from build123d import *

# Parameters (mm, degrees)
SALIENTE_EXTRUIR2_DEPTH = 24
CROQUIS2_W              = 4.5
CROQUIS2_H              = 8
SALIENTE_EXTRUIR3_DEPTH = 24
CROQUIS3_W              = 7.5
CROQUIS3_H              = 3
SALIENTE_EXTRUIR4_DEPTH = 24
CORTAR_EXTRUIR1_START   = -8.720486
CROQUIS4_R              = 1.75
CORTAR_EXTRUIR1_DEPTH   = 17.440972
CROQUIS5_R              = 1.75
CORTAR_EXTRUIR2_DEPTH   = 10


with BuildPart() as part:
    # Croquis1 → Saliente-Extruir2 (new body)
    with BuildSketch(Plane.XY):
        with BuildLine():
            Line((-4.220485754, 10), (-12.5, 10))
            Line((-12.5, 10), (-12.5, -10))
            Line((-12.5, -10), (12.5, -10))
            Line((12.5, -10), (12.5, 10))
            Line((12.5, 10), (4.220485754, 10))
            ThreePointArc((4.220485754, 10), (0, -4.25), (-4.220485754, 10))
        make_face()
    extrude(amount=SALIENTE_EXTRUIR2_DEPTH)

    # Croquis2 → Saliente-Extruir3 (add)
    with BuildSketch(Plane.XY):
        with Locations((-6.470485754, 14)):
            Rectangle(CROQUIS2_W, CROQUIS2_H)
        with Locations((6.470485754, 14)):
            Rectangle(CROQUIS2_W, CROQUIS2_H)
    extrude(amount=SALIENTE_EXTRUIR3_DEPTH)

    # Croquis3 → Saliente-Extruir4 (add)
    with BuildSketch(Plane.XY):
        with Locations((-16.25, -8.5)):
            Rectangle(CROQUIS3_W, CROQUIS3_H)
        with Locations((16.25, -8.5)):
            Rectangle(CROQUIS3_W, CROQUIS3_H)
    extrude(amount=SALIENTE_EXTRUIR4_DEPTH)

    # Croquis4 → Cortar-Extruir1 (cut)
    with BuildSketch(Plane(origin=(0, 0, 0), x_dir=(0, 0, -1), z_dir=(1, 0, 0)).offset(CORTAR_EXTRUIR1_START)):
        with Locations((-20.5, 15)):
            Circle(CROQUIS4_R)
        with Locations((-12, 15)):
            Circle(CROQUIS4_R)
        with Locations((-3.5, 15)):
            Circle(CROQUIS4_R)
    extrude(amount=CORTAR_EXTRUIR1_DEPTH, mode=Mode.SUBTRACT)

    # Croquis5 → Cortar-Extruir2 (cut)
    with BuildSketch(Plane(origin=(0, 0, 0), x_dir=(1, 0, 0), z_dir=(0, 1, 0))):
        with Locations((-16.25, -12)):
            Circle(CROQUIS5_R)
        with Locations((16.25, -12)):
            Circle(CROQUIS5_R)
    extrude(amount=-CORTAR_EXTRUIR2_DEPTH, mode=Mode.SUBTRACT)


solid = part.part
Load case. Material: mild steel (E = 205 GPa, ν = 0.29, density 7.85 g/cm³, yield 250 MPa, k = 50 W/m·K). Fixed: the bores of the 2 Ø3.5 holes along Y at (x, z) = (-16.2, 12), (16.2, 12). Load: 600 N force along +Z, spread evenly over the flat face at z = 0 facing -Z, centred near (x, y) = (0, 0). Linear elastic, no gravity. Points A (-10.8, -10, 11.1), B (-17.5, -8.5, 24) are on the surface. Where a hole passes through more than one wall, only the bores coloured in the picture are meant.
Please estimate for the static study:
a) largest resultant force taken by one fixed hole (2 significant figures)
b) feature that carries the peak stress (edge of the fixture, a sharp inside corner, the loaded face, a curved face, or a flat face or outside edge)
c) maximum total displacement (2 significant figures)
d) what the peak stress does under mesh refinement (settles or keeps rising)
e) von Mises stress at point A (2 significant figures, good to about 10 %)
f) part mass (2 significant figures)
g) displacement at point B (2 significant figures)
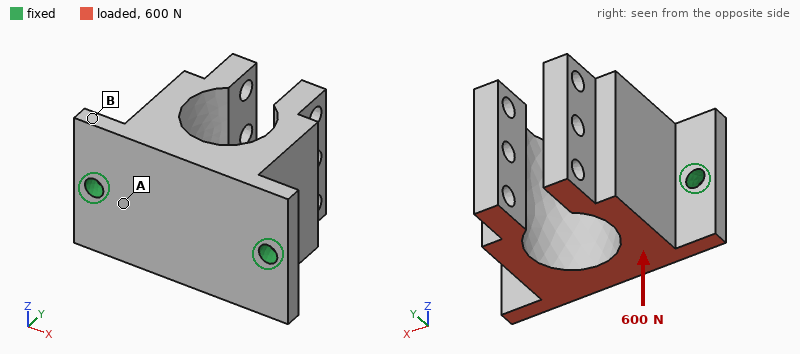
300 N
edge of the fixture
23 µm
keeps rising
17 MPa
80 g
7.4 µm
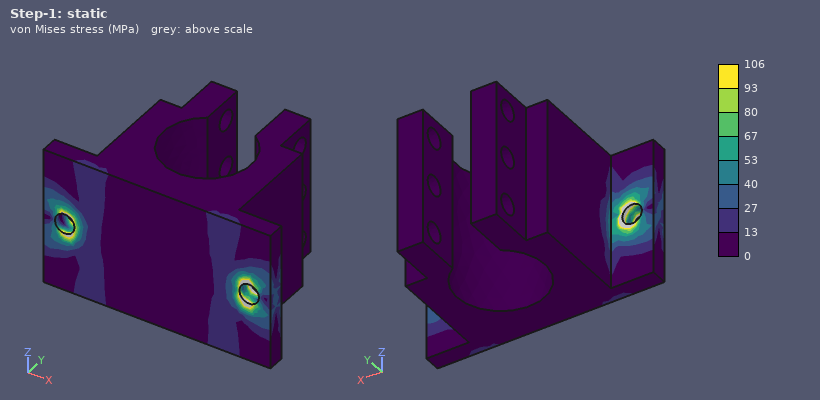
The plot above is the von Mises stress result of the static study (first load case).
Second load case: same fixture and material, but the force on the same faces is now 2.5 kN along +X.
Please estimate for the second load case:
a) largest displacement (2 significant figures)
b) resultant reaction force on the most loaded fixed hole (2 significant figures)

36 µm
1.7 kN
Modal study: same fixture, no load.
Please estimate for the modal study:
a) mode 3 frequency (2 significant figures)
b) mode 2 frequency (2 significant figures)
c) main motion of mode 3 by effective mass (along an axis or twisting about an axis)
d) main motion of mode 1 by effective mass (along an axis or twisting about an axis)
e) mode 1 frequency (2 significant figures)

8200 Hz
6800 Hz
along X
along Z
3400 Hz
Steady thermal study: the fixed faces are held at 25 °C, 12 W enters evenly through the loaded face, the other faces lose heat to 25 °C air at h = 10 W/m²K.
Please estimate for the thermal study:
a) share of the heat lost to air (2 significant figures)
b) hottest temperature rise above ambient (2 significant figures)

6.3 %
26 K
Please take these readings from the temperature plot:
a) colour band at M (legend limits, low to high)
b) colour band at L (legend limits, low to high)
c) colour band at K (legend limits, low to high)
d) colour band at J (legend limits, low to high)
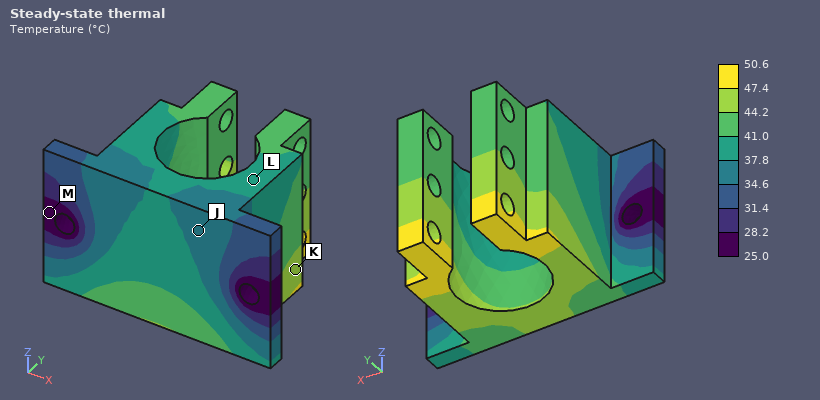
25.0 to 28.2 °C
37.8 to 41.0 °C
44.2 to 47.4 °C
34.6 to 37.8 °C
